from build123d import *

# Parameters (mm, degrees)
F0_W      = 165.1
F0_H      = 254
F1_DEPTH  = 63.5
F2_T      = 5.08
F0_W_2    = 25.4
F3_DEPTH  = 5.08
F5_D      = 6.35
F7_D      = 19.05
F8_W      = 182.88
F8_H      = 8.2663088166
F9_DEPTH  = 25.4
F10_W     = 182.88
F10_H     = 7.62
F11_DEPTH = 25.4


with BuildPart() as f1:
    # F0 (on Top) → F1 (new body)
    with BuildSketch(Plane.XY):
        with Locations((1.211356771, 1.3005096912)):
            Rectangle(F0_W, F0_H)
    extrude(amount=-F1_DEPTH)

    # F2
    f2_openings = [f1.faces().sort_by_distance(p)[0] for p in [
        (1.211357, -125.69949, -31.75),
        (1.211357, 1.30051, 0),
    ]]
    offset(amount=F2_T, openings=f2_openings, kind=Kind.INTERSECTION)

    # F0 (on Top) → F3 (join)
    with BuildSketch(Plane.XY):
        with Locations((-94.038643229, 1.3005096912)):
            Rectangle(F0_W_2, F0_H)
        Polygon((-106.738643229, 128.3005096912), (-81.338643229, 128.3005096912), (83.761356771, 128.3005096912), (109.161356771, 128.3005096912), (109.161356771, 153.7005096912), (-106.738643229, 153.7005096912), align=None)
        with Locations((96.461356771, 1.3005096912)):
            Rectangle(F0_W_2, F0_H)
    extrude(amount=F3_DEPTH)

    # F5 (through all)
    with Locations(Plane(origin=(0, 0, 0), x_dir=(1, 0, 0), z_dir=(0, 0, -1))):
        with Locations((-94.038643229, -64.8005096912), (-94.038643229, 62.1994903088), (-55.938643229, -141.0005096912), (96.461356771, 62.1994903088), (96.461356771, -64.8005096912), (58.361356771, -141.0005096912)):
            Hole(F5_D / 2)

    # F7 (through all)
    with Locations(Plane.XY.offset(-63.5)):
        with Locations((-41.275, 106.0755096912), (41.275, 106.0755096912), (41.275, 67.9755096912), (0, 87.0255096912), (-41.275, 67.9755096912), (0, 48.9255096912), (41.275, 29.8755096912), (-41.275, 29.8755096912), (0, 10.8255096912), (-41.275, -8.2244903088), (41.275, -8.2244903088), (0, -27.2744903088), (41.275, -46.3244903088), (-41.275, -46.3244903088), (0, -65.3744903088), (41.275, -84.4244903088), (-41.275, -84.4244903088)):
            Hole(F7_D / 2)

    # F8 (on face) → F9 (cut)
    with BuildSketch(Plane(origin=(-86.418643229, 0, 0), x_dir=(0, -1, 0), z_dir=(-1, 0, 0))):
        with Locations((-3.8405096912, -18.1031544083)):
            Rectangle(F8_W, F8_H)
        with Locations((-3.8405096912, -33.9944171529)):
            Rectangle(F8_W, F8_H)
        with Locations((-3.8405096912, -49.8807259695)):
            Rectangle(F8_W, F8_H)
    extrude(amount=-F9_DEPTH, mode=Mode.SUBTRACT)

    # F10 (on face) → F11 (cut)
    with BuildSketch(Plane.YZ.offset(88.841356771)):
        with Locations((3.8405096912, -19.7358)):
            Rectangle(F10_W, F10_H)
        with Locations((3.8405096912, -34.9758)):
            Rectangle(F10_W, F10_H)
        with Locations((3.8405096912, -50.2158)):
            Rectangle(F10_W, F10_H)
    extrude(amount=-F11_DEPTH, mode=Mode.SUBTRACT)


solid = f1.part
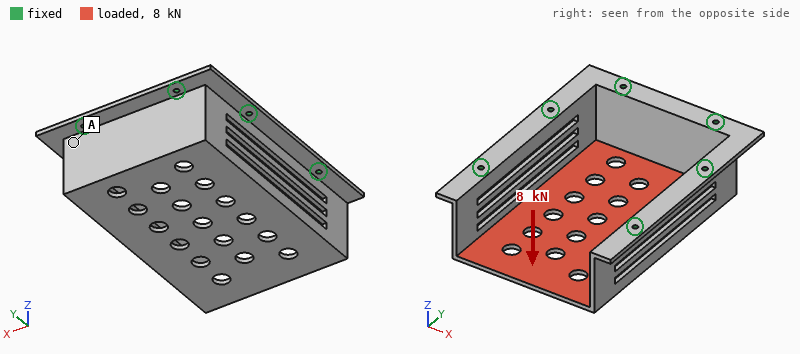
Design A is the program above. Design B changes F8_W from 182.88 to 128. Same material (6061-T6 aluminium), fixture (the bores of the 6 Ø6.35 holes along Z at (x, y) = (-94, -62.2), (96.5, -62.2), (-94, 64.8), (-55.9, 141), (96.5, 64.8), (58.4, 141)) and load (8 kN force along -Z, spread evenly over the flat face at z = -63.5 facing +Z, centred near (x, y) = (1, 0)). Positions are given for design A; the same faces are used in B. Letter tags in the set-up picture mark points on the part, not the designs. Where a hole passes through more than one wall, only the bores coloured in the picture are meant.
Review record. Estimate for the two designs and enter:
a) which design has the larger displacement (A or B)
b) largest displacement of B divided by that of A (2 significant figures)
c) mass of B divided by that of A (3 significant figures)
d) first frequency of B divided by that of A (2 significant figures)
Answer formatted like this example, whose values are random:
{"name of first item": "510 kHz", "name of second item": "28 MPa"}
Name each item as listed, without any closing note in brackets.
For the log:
{"which design has the larger displacement": "A", "largest displacement of B divided by that of A": "0.85", "mass of B divided by that of A": "1.01", "first frequency of B divided by that of A": "1.1"}
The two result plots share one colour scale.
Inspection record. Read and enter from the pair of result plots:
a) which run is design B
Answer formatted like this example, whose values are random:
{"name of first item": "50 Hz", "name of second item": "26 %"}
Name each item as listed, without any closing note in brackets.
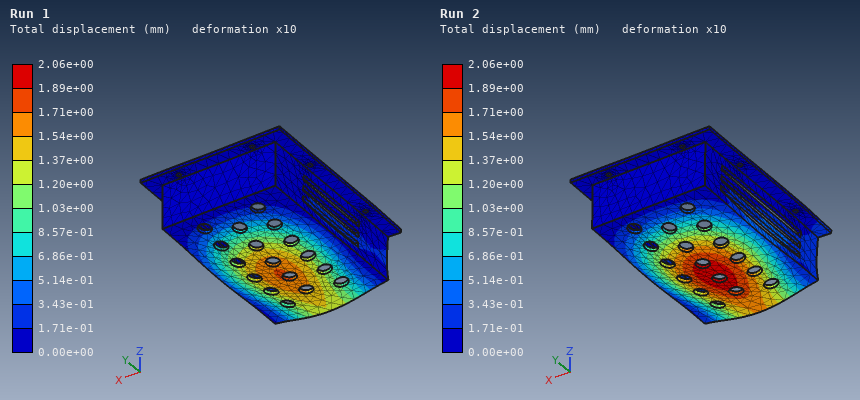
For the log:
{"which run is design B": "Run 1"}
